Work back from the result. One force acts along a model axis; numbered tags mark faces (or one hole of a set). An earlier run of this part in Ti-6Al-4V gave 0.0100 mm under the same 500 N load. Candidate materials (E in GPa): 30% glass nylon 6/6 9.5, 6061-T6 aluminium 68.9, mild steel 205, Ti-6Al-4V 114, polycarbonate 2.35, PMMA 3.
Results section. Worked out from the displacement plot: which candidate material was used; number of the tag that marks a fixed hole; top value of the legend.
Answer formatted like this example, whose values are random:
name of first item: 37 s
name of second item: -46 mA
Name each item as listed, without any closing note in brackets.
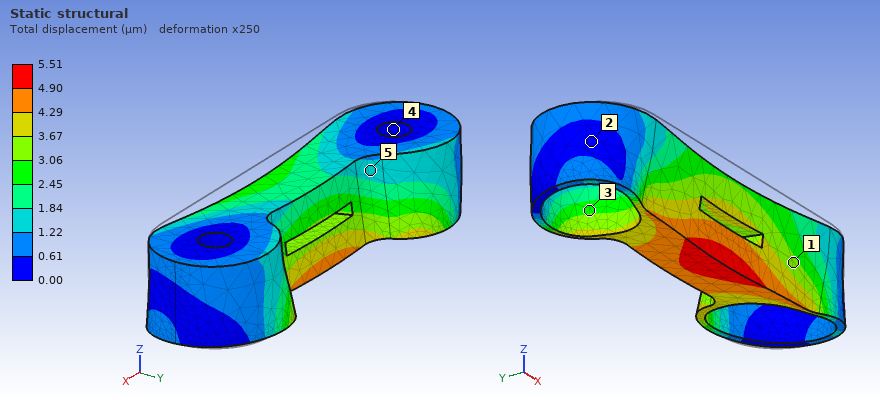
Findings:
which candidate material was used: mild steel
number of the tag that marks a fixed hole: 4
top value of the legend: 5.51 µm
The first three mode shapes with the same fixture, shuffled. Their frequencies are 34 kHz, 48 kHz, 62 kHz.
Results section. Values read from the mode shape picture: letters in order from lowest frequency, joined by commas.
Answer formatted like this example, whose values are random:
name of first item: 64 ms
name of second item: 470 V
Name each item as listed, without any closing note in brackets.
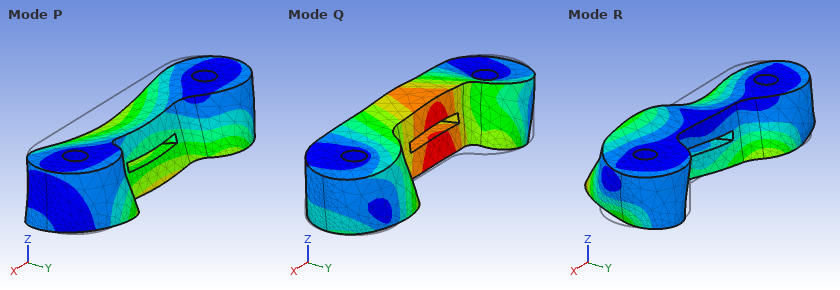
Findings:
letters in order from lowest frequency, joined by commas: P, Q, R
